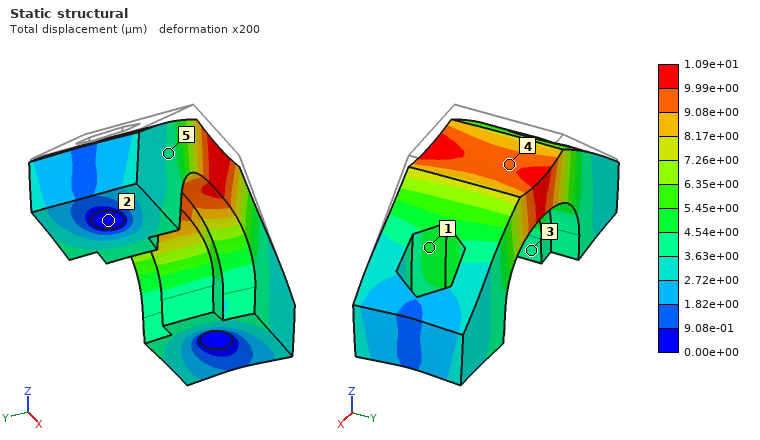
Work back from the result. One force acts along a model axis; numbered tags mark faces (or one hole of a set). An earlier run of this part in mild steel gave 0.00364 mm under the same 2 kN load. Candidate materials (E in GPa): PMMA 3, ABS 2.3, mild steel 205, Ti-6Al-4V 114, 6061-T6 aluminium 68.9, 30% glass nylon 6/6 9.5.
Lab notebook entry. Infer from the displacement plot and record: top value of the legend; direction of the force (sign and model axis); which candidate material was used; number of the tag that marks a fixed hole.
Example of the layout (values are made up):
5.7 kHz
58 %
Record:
1.09e+01 µm
-Z
6061-T6 aluminium
2
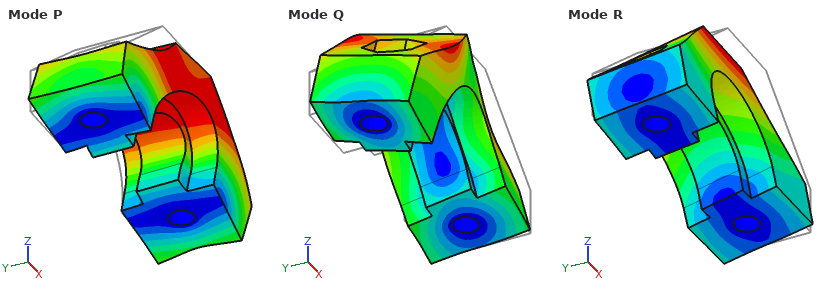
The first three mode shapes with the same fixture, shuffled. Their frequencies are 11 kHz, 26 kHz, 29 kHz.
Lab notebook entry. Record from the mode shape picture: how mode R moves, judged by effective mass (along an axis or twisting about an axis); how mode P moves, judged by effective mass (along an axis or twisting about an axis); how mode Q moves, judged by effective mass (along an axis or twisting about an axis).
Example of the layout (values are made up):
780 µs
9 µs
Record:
along Y
along X
twisting about Z
